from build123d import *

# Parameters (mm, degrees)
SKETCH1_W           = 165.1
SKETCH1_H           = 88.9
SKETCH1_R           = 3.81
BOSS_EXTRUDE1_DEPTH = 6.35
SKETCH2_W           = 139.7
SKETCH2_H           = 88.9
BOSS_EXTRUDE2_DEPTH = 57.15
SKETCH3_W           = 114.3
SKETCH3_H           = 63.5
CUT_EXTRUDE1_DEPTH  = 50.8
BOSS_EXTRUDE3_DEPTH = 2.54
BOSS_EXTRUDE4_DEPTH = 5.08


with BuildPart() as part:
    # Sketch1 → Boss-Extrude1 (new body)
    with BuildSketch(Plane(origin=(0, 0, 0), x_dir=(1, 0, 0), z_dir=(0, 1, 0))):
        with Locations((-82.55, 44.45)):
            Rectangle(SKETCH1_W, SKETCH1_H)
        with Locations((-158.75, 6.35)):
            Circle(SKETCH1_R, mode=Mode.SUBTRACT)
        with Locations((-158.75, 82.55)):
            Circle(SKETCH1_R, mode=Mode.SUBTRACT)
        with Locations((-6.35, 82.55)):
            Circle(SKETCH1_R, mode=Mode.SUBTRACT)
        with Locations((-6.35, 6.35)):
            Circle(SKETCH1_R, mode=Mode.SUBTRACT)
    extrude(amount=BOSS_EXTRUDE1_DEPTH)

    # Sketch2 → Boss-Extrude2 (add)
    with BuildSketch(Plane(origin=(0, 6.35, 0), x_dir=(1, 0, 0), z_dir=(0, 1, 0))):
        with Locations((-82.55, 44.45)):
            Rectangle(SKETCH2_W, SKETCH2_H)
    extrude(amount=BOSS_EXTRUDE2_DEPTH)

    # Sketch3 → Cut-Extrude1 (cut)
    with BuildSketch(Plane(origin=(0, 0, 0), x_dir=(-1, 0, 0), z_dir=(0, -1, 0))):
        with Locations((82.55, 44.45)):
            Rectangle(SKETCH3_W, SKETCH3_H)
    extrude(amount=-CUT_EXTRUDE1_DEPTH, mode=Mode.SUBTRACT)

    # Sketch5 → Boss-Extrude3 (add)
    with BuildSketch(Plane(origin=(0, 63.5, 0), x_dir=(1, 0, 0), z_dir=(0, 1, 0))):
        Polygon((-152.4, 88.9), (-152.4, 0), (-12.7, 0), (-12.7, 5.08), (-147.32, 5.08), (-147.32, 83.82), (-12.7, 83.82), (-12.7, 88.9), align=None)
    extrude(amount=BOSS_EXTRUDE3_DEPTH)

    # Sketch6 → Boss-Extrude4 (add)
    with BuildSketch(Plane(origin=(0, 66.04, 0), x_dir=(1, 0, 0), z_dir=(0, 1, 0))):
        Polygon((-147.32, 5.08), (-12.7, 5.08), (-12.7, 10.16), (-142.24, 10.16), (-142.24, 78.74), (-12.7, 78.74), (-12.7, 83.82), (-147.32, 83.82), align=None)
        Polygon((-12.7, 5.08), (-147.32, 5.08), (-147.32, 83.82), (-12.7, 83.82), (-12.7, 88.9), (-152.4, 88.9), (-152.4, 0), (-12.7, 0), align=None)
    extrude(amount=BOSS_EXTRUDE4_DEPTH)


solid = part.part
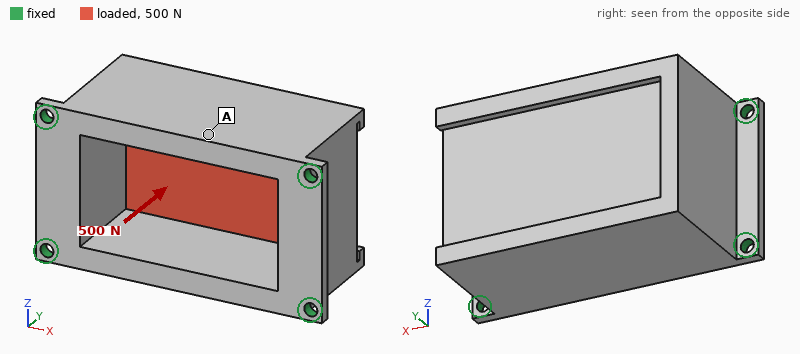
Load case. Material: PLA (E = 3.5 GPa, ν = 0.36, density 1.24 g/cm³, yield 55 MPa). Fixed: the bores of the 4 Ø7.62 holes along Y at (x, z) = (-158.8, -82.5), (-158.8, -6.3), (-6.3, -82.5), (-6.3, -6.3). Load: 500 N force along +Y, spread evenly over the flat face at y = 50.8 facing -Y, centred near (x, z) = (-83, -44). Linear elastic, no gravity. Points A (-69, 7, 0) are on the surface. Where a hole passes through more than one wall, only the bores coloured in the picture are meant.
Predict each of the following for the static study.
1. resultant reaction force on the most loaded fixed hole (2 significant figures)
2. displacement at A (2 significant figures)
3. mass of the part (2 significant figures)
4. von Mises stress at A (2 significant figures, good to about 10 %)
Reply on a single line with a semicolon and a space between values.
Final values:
150 N; 19 µm; 570 g; 0.25 MPa
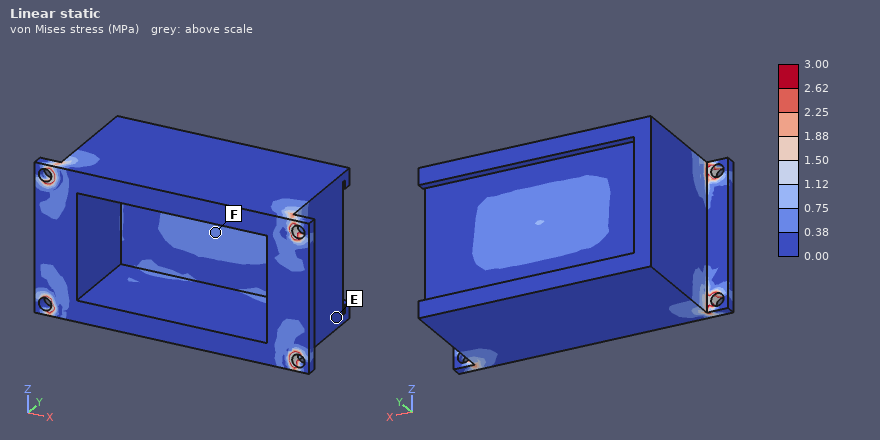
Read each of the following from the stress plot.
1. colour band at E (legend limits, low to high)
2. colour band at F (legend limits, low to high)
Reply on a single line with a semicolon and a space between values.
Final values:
0.00 to 0.38 MPa; 0.38 to 0.75 MPa
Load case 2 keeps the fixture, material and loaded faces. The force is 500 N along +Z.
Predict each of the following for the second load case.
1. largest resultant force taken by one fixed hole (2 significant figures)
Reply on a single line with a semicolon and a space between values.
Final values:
210 N
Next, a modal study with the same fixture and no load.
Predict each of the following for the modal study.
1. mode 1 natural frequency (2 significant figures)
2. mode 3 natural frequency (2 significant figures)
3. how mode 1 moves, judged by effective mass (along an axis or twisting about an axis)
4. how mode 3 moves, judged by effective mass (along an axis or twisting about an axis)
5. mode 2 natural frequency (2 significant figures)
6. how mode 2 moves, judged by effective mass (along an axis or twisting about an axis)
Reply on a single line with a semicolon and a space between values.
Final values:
850 Hz; 1400 Hz; along Z; along X; 1200 Hz; along Y
